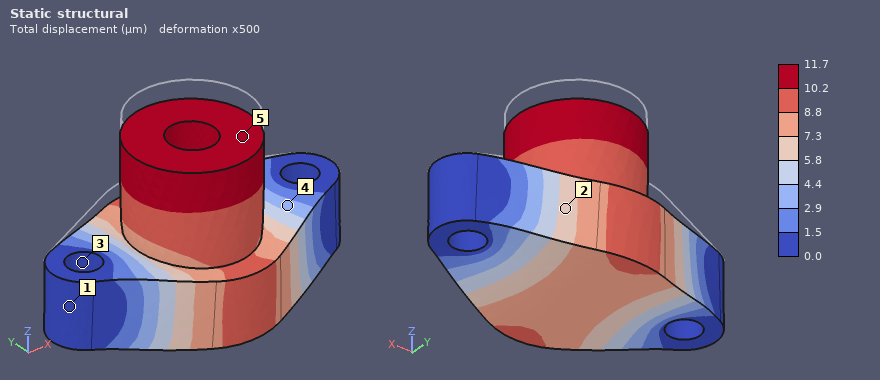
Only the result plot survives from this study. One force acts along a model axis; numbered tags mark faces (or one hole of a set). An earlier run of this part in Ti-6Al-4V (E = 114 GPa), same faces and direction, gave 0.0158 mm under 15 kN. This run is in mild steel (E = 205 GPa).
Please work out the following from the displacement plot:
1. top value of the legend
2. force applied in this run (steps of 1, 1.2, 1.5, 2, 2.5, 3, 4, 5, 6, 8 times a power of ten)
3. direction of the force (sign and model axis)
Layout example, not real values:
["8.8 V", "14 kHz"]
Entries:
["11.7 µm", "20 kN", "-Z"]
